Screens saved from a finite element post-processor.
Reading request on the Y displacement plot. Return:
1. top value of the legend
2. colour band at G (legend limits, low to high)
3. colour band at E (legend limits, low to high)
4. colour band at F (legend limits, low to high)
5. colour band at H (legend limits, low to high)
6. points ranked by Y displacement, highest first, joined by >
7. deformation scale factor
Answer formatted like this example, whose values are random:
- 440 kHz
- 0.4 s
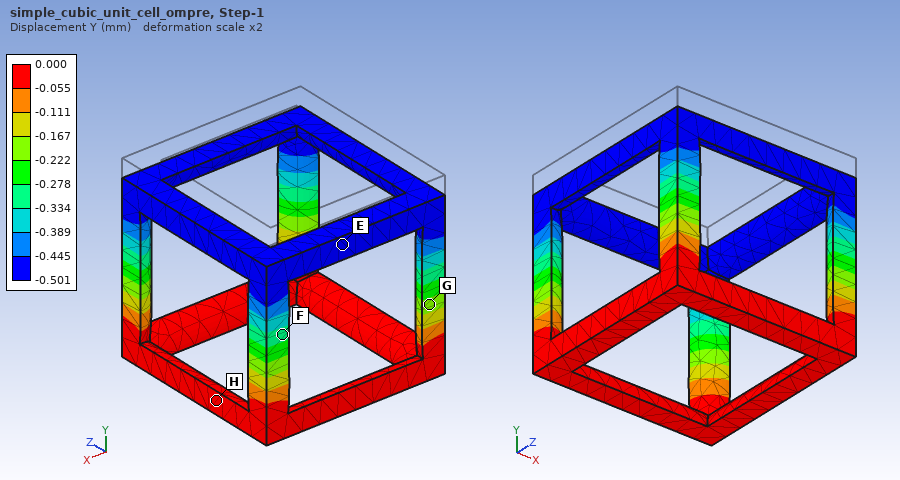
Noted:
- 0.000 mm
- -0.222 to -0.167 mm
- -0.501 to -0.445 mm
- -0.334 to -0.278 mm
- -0.055 to 0.000 mm
- H > G > F > E
- 2
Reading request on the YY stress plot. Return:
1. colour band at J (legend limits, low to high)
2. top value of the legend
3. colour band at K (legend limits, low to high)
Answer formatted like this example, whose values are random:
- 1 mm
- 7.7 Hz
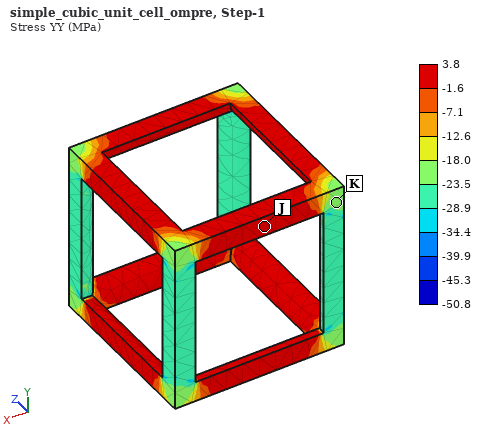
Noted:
- -1.6 to 3.8 MPa
- 3.8 MPa
- -23.5 to -18.0 MPa
